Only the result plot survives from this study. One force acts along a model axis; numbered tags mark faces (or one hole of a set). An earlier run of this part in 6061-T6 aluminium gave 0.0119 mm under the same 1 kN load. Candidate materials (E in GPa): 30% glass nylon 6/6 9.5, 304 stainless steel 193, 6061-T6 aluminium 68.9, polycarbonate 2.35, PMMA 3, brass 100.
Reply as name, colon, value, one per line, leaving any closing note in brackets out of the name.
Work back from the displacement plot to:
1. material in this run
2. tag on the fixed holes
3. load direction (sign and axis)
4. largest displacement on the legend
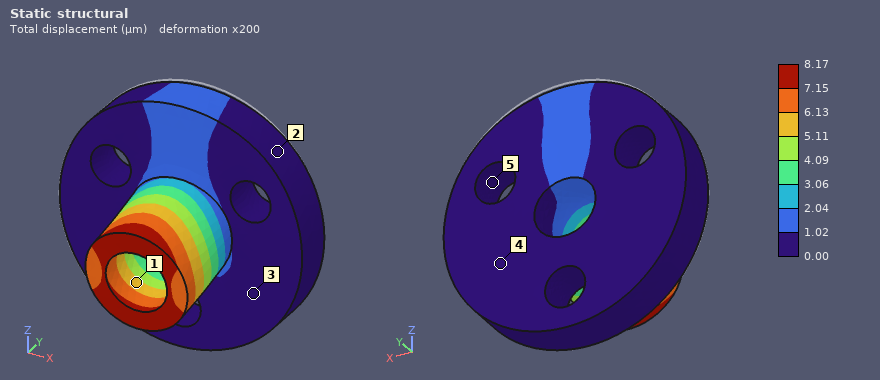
material in this run: brass
tag on the fixed holes: 5
load direction: -Z
largest displacement on the legend: 8.17 µm
